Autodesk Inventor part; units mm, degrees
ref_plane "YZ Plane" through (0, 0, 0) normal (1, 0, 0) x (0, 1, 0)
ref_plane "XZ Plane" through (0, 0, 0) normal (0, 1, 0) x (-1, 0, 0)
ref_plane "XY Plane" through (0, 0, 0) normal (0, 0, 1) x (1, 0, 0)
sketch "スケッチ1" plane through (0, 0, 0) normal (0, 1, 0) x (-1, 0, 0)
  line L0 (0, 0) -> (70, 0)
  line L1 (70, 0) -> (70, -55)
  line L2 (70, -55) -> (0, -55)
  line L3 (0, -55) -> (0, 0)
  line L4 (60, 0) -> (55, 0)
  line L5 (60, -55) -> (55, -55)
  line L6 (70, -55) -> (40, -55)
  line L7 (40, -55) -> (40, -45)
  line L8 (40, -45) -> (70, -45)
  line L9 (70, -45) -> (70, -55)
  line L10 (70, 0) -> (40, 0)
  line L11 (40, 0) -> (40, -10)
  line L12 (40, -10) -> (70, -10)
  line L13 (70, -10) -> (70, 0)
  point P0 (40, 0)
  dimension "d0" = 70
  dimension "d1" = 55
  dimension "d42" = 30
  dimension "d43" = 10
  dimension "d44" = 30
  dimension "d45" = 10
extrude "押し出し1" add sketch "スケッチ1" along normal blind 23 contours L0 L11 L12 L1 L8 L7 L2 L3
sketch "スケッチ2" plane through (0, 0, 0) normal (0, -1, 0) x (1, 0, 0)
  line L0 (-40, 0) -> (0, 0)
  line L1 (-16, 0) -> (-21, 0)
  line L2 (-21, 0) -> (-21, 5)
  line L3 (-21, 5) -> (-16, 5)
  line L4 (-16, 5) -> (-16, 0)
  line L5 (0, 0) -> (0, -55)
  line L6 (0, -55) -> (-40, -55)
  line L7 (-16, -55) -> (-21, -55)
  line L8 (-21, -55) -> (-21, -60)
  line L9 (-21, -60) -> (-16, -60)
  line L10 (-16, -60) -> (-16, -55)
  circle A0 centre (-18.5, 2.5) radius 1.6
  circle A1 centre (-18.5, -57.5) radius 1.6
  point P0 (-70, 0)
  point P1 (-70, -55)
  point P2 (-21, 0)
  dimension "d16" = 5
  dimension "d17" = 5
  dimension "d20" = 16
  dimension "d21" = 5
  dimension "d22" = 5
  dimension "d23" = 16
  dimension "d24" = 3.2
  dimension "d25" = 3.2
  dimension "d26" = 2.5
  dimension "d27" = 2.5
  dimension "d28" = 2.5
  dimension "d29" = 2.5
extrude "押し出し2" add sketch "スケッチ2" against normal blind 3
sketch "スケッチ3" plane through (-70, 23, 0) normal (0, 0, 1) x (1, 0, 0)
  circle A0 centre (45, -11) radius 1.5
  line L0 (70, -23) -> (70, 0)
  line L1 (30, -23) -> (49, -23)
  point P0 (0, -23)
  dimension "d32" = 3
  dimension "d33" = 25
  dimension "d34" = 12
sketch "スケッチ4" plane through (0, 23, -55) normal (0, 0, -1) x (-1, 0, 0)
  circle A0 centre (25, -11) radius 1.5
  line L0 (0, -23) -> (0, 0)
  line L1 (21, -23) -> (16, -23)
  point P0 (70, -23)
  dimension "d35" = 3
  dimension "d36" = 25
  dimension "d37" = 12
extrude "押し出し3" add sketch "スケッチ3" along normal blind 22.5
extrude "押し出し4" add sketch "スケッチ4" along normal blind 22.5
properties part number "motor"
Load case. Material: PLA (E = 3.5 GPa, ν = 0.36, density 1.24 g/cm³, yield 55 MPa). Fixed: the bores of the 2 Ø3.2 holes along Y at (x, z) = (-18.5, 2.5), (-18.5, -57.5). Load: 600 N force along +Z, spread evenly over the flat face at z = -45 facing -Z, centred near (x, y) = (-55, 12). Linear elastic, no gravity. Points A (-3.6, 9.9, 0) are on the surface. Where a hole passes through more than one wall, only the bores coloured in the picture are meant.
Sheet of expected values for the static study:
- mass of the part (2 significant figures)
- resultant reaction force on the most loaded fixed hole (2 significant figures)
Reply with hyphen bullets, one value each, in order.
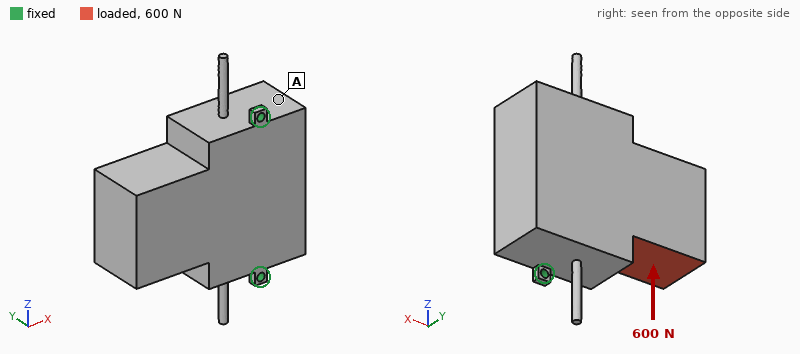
- 93 g
- 500 N
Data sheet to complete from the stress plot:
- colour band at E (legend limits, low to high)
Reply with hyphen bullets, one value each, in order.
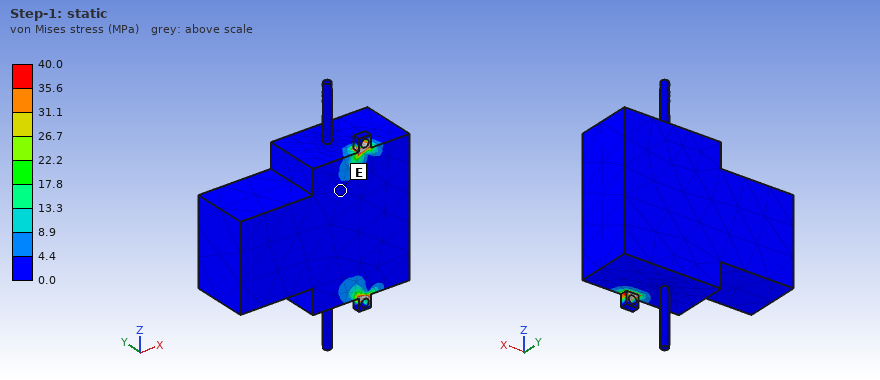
- 0.0 to 4.4 MPa
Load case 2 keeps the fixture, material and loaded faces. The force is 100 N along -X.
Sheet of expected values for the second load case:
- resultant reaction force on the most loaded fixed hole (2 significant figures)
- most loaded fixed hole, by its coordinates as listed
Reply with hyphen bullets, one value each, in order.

- 81 N
- (-18.5, -57.5)
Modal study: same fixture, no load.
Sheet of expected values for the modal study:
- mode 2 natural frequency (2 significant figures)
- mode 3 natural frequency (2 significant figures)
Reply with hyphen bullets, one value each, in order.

- 1300 Hz
- 1300 Hz
